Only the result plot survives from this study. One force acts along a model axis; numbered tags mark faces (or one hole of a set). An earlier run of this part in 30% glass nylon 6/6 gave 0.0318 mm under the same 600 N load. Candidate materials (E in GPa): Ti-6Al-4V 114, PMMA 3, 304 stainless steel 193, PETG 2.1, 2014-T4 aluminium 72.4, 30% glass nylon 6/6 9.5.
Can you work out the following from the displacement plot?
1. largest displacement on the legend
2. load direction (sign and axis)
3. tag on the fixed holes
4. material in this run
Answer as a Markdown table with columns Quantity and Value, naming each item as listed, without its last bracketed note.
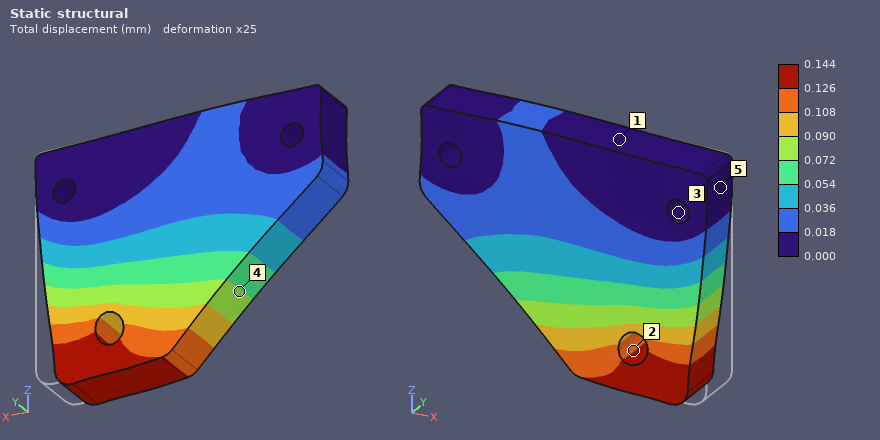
| Quantity | Value |
|---|---|
| largest displacement on the legend | 0.144 mm |
| load direction | -X |
| tag on the fixed holes | 3 |
| material in this run | PETG |
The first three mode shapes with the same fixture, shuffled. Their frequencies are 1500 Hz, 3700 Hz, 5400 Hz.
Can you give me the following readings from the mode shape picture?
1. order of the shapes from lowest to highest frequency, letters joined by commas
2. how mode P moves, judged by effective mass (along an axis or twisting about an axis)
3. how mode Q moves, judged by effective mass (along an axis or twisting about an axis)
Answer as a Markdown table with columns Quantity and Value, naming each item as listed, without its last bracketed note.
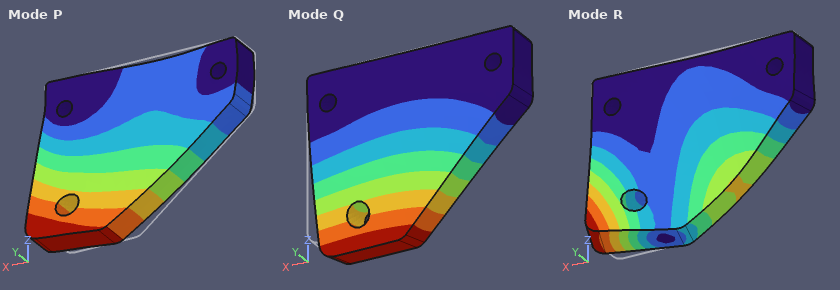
| Quantity | Value |
|---|---|
| order of the shapes from lowest to highest frequency, letters joined by commas | Q, R, P |
| how mode P moves, judged by effective mass | along X |
| how mode Q moves, judged by effective mass | along Y |
